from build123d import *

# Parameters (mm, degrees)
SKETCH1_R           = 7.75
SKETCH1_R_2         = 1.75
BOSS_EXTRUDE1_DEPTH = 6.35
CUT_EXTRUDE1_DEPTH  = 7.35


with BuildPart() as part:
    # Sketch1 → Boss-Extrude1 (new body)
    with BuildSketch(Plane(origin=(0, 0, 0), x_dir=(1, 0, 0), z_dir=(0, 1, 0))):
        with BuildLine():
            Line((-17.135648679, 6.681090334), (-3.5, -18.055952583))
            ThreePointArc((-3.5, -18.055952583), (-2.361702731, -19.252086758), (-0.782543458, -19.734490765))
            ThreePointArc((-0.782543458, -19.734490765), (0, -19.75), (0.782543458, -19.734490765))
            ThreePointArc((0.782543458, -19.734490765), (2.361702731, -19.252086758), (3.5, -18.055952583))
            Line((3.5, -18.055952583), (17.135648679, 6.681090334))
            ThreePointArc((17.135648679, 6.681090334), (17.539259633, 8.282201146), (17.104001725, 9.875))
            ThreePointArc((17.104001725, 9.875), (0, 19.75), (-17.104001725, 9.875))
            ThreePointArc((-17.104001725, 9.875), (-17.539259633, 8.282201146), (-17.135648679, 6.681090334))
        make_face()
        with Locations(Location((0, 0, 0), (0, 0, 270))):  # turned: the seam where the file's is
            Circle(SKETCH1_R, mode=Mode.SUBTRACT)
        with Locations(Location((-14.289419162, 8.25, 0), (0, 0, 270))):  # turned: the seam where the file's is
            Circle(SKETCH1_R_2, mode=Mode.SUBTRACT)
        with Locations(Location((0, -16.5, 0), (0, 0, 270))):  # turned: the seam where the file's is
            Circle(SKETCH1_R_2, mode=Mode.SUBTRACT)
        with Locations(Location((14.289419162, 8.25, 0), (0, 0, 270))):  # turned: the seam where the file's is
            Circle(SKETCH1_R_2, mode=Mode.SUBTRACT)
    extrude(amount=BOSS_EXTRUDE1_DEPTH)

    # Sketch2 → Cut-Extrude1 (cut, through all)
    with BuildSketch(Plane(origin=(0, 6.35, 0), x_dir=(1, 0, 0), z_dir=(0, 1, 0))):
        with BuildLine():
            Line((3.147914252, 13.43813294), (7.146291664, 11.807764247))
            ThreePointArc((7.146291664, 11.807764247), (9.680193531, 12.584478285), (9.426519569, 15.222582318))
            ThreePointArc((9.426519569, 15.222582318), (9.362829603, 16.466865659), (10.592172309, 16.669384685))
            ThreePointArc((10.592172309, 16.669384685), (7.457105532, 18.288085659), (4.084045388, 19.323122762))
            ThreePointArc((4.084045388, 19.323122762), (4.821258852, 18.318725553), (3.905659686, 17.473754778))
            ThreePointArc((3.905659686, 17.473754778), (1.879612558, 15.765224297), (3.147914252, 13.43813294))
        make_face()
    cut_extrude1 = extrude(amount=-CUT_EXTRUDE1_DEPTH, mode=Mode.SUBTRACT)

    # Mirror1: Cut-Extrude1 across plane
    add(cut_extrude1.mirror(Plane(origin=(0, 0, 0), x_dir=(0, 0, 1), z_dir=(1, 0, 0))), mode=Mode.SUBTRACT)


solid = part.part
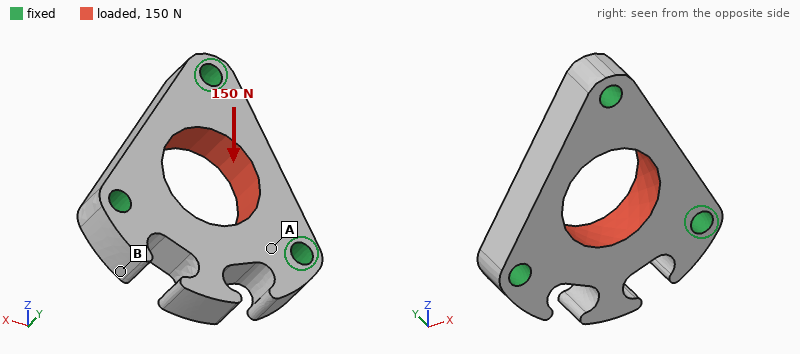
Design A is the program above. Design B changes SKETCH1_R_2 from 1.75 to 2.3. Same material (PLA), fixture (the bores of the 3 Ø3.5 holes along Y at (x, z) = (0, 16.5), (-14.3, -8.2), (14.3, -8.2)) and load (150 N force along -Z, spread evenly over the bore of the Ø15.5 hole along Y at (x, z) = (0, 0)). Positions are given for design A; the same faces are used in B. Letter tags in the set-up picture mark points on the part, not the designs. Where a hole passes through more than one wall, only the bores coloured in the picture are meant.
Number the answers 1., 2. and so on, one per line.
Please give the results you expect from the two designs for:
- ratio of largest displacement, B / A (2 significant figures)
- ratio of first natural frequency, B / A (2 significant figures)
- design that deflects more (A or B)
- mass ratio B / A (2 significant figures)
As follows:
1. 0.83
2. 1.0
3. A
4. 0.96
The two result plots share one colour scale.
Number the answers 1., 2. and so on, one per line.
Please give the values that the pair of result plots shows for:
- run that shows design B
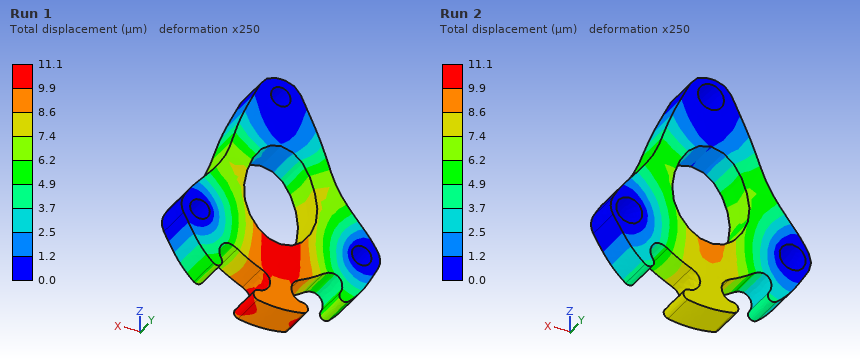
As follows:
1. Run 2
